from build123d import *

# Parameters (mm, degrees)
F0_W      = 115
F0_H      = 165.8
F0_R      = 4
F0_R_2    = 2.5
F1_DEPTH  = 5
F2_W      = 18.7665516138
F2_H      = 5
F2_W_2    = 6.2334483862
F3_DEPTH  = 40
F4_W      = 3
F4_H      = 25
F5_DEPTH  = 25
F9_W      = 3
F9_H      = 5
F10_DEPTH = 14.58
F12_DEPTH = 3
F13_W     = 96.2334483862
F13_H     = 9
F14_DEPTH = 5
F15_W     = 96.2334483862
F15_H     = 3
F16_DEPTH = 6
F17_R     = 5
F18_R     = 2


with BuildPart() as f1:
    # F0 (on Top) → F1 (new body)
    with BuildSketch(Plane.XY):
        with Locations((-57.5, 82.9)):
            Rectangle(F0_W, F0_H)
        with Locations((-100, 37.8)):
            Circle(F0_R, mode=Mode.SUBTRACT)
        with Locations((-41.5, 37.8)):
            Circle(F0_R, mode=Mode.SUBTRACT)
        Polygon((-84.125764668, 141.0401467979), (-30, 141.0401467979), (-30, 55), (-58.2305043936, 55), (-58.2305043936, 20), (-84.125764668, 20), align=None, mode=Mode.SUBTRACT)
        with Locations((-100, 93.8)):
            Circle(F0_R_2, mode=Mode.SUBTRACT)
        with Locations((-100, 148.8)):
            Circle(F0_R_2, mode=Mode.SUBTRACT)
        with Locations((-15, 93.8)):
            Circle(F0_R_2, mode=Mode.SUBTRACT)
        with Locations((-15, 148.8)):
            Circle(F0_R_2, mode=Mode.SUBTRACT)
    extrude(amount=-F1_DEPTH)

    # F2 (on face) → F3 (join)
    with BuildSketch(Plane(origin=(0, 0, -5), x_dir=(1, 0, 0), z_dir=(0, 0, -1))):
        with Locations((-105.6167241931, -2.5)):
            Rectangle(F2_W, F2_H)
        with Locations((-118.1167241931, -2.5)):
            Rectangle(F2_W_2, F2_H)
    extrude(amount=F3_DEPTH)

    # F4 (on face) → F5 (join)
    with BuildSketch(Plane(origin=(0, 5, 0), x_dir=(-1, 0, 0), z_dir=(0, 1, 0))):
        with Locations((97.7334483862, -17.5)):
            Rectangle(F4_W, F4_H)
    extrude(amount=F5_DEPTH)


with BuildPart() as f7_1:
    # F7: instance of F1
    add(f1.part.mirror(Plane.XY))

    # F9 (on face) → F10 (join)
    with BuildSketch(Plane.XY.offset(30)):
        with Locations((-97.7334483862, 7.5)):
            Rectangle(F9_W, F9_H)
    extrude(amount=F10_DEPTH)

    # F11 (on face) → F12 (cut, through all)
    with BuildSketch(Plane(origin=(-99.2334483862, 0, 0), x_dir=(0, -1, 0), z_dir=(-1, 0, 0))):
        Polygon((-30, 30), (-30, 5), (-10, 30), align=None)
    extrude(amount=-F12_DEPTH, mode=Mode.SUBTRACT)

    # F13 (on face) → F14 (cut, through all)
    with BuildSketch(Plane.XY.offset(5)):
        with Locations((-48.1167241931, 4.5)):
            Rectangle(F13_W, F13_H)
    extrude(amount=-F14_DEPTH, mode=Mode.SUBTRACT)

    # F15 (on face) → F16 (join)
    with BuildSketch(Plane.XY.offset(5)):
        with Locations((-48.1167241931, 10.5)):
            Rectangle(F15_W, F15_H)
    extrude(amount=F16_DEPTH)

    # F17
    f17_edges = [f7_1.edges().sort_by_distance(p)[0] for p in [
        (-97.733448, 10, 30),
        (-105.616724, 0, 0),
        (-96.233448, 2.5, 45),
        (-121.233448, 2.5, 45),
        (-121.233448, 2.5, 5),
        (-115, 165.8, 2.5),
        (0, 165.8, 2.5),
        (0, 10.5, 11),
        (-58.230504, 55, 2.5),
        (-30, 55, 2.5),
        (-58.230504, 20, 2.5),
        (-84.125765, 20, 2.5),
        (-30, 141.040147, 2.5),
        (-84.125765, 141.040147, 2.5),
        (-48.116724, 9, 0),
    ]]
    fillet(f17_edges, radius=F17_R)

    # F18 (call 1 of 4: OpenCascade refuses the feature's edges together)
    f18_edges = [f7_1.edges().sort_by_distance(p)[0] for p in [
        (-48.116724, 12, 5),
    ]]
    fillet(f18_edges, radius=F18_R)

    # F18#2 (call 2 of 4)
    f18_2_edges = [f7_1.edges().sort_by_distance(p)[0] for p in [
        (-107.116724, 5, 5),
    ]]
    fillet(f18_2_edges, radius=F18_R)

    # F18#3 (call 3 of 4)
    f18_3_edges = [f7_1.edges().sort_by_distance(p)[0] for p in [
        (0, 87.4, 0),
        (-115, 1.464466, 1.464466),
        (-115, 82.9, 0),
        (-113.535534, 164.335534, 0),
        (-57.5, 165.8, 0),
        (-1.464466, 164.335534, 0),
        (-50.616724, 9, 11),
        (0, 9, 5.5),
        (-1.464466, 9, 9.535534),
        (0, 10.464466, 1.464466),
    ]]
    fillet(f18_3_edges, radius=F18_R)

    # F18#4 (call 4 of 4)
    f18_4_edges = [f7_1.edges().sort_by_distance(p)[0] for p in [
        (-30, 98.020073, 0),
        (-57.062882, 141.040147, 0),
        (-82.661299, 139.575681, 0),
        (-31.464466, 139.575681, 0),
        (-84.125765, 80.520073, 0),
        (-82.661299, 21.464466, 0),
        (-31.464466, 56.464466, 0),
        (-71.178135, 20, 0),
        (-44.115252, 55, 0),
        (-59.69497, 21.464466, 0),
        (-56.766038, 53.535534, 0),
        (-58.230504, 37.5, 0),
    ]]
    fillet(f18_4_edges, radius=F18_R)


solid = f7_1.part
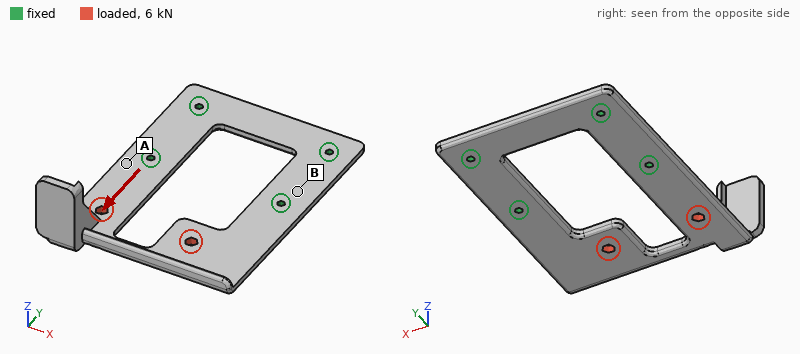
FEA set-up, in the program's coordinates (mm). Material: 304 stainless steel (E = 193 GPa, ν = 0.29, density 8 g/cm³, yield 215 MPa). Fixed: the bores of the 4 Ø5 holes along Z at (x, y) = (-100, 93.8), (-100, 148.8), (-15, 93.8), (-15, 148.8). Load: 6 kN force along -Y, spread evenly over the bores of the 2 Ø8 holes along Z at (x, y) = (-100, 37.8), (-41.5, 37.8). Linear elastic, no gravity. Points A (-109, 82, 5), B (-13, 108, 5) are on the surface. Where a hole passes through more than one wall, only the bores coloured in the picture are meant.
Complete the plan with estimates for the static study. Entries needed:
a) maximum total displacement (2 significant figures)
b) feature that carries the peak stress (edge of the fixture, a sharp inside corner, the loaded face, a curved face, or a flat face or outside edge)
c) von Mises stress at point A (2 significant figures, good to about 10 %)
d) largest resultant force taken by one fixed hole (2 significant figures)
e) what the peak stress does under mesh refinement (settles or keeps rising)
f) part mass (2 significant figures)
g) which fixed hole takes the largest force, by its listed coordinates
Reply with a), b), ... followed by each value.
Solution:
a) 35 µm
b) a sharp inside corner
c) 30 MPa
d) 3.3 kN
e) keeps rising
f) 550 g
g) (-100, 93.8)
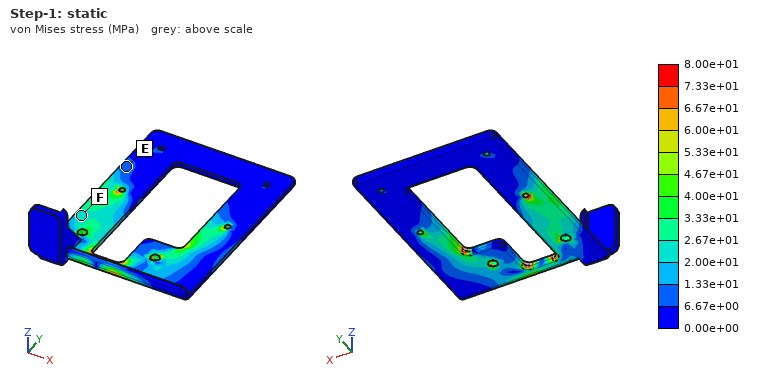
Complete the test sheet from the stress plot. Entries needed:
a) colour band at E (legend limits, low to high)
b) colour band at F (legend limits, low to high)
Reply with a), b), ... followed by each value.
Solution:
a) 6.67e+00 to 1.33e+01 MPa
b) 2.00e+01 to 2.67e+01 MPa
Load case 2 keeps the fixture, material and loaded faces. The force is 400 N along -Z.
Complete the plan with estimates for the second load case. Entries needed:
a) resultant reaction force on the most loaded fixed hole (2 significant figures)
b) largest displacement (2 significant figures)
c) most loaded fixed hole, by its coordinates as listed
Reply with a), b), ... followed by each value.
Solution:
a) 270 N
b) 0.51 mm
c) (-100, 93.8)
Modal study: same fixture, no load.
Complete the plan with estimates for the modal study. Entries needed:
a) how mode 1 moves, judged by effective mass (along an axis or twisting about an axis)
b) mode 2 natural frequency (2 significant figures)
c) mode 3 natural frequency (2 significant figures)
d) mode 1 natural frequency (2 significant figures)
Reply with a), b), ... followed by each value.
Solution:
a) along Z
b) 630 Hz
c) 1600 Hz
d) 290 Hz
